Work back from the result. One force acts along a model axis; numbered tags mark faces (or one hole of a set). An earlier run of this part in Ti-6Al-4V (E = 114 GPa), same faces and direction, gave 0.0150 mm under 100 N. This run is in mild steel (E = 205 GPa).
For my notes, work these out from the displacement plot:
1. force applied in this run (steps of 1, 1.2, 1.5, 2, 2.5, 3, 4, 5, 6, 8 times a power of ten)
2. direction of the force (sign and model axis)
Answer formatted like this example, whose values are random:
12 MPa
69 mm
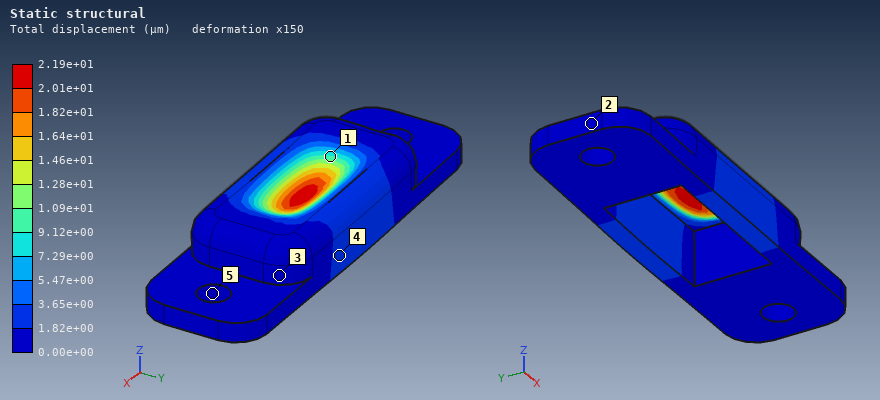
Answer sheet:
250 N
-Z
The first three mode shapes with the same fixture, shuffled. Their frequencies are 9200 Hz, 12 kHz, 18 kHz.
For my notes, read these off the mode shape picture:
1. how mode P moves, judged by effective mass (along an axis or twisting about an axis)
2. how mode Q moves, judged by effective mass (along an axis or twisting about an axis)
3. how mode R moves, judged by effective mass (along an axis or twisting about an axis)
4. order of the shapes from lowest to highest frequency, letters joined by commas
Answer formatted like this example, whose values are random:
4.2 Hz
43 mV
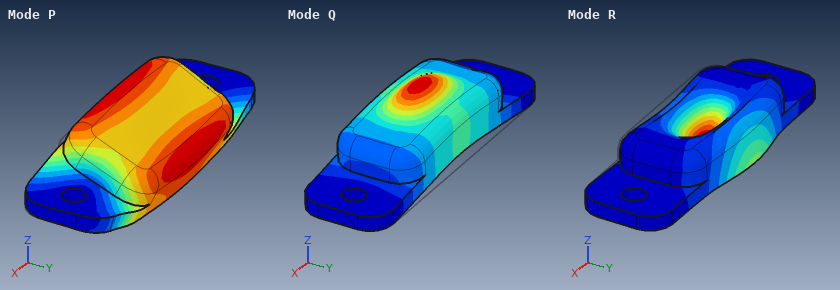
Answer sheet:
along Y
along Z
along Y
P, Q, R
